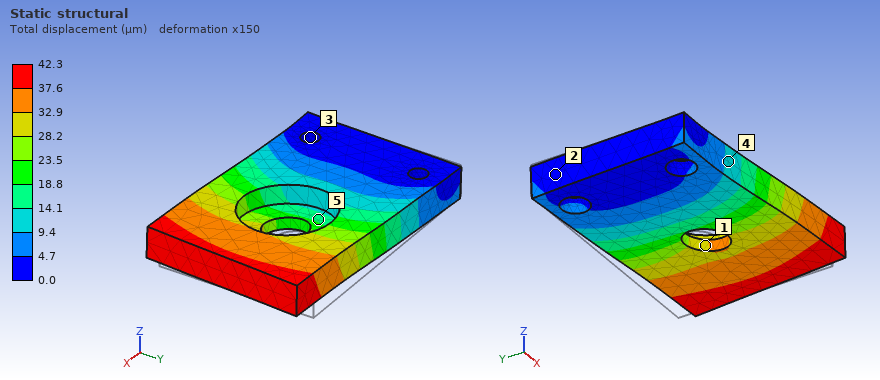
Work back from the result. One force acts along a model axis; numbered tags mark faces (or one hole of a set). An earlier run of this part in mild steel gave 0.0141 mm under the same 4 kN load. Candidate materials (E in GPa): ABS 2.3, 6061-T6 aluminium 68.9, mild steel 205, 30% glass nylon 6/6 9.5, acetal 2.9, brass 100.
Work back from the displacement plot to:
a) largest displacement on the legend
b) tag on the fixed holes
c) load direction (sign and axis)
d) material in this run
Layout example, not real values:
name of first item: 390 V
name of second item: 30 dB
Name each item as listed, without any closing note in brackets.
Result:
largest displacement on the legend: 42.3 µm
tag on the fixed holes: 3
load direction: -Y
material in this run: 6061-T6 aluminium
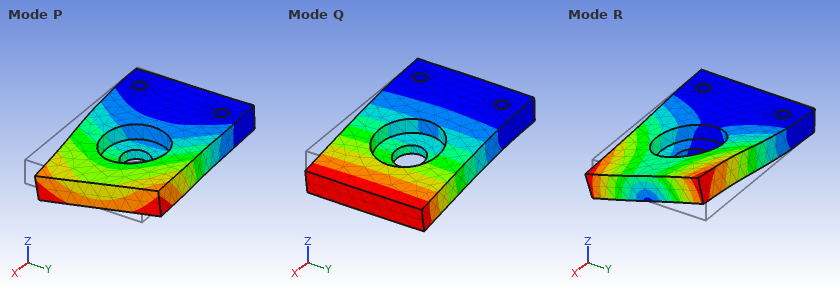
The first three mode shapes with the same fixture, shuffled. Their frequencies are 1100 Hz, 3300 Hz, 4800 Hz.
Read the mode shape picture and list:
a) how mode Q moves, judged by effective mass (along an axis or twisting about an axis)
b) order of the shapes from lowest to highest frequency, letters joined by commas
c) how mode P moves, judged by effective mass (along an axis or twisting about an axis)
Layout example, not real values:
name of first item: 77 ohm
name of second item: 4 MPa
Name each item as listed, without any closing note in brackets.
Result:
how mode Q moves, judged by effective mass: along Z
order of the shapes from lowest to highest frequency, letters joined by commas: Q, R, P
how mode P moves, judged by effective mass: along Y
